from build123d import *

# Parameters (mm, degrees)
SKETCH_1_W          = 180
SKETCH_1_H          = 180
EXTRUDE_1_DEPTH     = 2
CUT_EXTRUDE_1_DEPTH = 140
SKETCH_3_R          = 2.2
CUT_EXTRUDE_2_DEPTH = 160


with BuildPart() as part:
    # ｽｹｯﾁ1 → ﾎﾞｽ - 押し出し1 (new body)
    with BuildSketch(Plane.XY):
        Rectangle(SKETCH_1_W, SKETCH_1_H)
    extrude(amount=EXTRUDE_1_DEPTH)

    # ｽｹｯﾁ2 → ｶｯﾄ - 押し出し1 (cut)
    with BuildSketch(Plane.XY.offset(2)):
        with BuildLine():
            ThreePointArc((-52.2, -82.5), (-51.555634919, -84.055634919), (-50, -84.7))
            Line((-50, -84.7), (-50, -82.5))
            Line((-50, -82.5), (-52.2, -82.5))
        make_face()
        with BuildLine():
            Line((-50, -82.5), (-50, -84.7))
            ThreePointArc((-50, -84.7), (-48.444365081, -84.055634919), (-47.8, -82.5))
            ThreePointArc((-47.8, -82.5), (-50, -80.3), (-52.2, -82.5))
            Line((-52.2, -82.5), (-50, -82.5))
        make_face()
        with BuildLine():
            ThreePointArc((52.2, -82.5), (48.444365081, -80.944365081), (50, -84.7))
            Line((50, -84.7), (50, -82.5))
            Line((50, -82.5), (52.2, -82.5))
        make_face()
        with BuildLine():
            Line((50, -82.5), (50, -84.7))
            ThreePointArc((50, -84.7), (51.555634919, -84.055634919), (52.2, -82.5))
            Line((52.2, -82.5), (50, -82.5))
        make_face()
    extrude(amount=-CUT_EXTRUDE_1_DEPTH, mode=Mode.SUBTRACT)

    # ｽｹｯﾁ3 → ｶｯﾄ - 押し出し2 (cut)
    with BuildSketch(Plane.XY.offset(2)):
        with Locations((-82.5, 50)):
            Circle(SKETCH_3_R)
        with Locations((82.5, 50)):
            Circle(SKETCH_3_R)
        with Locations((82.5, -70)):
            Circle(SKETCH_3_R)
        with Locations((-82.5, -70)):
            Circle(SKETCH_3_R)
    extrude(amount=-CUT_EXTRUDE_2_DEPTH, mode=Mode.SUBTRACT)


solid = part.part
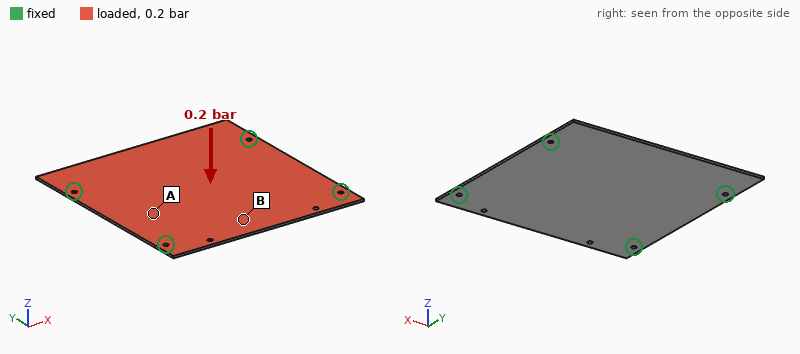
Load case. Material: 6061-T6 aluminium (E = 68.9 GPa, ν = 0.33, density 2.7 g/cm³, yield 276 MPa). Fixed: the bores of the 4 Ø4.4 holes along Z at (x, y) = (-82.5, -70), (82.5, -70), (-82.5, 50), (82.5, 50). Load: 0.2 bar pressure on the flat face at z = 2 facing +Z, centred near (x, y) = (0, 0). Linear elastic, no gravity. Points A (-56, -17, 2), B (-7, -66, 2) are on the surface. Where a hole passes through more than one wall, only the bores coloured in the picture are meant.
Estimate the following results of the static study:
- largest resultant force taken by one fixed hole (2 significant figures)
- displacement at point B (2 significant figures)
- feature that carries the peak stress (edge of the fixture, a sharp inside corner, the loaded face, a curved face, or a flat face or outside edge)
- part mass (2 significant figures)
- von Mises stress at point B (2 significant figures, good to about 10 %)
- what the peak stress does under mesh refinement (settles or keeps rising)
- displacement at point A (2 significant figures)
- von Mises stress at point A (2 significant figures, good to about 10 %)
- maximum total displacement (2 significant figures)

180 N
1.2 mm
edge of the fixture
170 g
40 MPa
keeps rising
0.77 mm
22 MPa
1.4 mm
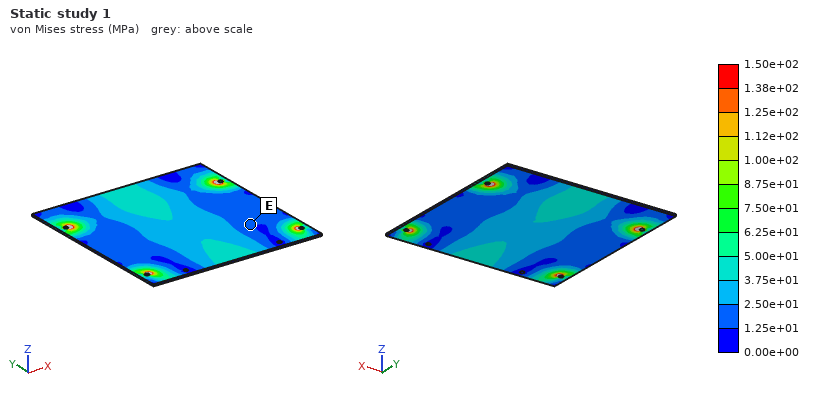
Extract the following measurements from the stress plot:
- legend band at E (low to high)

1.25e+01 to 2.50e+01 MPa
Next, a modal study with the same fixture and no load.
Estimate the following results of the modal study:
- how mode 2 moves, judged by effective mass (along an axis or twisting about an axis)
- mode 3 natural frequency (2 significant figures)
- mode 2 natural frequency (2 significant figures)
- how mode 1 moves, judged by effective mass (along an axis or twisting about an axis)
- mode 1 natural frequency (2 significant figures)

twisting about X
540 Hz
370 Hz
along Z
300 Hz
